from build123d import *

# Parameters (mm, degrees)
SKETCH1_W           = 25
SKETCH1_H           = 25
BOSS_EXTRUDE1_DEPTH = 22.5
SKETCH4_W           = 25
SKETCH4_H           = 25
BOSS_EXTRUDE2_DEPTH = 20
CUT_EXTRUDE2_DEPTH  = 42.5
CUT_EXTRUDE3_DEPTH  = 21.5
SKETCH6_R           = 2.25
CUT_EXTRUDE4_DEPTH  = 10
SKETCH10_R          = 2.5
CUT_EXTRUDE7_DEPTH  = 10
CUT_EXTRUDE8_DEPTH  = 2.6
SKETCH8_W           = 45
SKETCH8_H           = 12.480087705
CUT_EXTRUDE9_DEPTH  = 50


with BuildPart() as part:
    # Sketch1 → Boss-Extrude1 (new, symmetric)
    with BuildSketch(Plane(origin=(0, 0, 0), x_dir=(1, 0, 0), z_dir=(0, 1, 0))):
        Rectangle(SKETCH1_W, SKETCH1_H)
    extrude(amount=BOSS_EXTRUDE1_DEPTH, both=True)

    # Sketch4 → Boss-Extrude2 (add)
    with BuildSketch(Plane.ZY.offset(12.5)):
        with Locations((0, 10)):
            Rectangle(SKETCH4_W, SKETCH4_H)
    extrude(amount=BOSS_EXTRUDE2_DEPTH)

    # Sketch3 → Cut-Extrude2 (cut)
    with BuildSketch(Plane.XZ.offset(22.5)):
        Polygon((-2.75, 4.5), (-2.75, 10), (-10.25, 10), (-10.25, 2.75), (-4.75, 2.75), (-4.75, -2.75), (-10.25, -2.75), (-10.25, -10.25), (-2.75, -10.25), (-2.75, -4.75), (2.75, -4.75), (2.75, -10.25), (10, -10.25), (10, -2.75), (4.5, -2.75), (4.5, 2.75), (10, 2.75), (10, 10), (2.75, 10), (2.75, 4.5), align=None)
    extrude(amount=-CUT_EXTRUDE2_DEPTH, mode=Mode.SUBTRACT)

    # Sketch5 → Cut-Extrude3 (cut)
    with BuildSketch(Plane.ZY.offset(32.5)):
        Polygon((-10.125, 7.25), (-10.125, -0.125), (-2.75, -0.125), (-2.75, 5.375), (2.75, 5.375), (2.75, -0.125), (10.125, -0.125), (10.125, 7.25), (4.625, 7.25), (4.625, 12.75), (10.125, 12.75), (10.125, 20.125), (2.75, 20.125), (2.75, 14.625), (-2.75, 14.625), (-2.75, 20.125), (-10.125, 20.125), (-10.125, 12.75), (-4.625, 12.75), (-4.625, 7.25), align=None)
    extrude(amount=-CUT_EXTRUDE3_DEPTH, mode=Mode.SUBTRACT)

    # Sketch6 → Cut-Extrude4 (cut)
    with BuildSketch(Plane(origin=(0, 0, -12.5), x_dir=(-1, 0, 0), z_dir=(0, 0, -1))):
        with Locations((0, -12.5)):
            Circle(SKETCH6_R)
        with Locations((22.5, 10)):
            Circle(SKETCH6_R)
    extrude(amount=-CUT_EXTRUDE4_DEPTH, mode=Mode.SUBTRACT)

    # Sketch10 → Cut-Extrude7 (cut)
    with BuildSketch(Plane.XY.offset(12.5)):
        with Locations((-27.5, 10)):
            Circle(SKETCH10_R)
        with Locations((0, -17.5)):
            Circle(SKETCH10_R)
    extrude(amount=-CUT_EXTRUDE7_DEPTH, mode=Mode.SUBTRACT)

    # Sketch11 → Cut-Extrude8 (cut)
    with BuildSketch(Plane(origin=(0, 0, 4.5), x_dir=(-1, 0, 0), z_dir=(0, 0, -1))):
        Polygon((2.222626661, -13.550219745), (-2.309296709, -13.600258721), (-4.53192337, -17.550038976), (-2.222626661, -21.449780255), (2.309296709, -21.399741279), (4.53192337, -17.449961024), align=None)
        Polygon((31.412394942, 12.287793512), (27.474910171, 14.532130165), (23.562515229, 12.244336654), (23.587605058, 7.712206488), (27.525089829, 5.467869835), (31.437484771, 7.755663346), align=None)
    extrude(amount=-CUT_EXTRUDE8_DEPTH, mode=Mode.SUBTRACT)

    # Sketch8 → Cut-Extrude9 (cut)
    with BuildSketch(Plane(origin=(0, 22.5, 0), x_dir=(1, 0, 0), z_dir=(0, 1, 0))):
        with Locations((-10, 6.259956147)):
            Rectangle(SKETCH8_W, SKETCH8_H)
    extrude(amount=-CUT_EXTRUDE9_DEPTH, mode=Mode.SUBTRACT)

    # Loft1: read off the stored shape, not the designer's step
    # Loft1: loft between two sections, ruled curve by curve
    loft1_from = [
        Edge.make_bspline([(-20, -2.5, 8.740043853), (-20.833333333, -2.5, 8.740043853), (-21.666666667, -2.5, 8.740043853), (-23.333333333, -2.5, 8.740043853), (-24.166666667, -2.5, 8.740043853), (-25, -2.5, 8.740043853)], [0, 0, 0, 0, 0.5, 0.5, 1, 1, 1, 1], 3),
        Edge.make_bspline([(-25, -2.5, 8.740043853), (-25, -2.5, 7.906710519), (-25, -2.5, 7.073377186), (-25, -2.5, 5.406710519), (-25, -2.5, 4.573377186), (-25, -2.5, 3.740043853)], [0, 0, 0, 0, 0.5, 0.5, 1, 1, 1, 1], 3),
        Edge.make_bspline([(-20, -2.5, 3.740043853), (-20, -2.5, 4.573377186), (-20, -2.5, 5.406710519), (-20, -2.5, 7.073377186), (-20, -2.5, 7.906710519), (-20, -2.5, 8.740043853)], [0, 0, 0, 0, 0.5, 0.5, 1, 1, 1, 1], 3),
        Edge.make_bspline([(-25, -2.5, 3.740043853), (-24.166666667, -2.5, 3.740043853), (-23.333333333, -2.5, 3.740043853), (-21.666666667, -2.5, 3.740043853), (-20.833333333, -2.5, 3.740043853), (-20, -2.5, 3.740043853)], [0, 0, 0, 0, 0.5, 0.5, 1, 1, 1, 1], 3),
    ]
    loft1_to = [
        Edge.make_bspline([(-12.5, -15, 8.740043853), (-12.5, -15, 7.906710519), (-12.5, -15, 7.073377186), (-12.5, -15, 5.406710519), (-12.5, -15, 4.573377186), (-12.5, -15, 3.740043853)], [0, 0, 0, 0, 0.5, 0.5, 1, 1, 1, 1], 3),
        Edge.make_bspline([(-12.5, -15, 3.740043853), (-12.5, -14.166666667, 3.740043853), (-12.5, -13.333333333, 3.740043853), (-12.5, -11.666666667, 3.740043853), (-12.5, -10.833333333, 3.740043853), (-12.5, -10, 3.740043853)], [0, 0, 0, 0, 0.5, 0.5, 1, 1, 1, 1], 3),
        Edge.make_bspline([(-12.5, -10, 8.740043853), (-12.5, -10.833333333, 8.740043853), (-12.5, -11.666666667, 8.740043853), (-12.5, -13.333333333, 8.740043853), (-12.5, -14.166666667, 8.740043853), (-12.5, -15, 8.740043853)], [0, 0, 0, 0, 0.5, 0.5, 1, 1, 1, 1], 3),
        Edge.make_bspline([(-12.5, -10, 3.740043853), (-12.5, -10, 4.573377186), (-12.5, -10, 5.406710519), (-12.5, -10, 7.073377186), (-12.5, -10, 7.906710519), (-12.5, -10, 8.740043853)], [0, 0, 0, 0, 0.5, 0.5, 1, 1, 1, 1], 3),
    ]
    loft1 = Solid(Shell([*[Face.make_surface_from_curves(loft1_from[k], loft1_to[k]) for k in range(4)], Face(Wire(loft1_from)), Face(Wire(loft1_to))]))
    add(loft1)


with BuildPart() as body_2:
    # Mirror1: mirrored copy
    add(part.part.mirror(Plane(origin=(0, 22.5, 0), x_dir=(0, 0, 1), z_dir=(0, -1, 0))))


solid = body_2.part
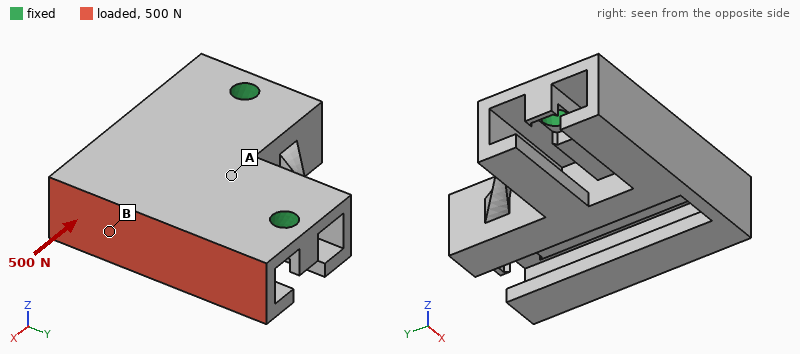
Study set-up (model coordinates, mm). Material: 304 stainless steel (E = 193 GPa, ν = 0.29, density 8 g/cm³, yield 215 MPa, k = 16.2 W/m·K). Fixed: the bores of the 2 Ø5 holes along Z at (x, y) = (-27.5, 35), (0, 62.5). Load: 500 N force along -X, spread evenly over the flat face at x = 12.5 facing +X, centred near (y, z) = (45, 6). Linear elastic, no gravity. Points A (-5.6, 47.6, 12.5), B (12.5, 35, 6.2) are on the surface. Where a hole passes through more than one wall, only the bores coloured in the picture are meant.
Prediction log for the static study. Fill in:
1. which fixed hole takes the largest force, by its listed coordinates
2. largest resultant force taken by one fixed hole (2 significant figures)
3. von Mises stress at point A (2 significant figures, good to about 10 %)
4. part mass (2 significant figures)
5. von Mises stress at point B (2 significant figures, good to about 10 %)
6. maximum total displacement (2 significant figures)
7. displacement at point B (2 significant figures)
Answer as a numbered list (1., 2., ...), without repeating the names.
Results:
1. (-27.5, 35)
2. 270 N
3. 5.2 MPa
4. 87 g
5. 14 MPa
6. 22 µm
7. 12 µm
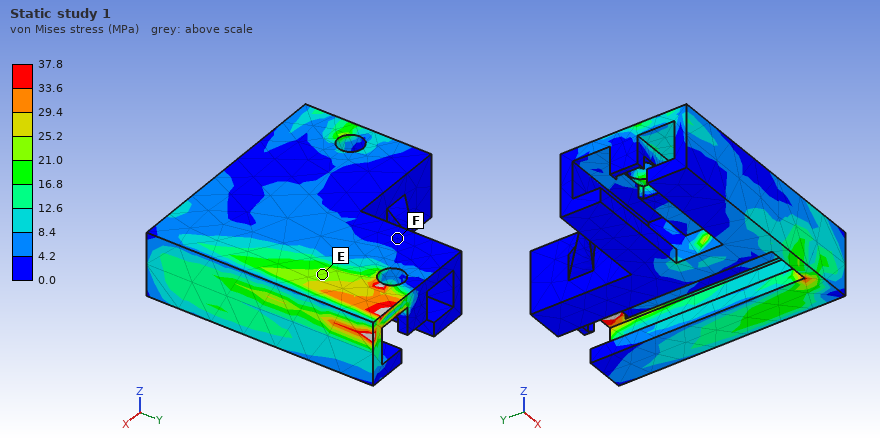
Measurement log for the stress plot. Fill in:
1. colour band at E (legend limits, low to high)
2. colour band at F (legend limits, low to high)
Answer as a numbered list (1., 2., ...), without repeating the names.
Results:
1. 21.0 to 25.2 MPa
2. 0.0 to 4.2 MPa
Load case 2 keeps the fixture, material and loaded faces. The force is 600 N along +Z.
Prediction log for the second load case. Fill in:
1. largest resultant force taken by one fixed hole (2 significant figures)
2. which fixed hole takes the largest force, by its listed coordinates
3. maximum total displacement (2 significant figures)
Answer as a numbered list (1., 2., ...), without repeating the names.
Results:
1. 530 N
2. (0, 62.5)
3. 69 µm
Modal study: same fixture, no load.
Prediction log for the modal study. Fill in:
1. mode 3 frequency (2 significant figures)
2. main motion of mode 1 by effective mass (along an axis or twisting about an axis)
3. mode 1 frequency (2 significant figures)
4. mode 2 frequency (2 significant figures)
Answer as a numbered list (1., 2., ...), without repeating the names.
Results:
1. 8600 Hz
2. along Z
3. 3000 Hz
4. 6300 Hz
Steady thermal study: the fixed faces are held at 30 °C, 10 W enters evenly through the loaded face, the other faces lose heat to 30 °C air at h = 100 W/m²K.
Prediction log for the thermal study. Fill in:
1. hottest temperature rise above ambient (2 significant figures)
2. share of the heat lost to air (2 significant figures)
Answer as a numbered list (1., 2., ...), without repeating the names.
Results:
1. 41 K
2. 78 %
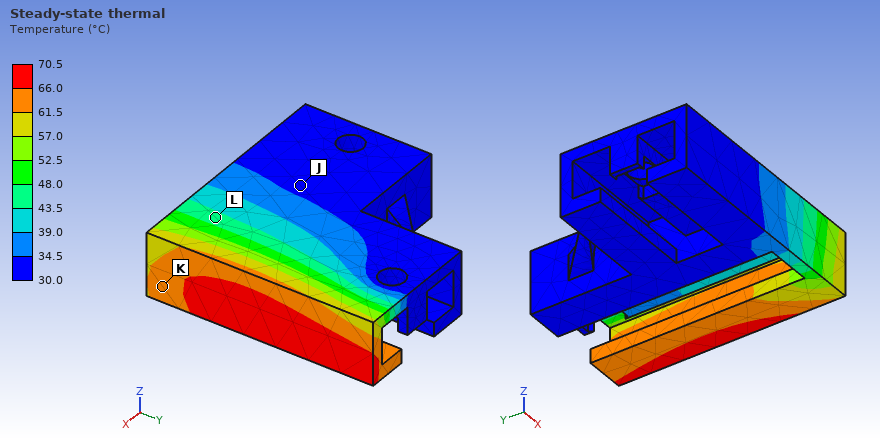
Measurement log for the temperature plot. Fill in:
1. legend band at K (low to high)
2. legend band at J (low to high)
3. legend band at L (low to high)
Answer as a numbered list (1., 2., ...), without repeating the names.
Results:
1. 61.5 to 66.0 °C
2. 30.0 to 34.5 °C
3. 43.5 to 48.0 °C
